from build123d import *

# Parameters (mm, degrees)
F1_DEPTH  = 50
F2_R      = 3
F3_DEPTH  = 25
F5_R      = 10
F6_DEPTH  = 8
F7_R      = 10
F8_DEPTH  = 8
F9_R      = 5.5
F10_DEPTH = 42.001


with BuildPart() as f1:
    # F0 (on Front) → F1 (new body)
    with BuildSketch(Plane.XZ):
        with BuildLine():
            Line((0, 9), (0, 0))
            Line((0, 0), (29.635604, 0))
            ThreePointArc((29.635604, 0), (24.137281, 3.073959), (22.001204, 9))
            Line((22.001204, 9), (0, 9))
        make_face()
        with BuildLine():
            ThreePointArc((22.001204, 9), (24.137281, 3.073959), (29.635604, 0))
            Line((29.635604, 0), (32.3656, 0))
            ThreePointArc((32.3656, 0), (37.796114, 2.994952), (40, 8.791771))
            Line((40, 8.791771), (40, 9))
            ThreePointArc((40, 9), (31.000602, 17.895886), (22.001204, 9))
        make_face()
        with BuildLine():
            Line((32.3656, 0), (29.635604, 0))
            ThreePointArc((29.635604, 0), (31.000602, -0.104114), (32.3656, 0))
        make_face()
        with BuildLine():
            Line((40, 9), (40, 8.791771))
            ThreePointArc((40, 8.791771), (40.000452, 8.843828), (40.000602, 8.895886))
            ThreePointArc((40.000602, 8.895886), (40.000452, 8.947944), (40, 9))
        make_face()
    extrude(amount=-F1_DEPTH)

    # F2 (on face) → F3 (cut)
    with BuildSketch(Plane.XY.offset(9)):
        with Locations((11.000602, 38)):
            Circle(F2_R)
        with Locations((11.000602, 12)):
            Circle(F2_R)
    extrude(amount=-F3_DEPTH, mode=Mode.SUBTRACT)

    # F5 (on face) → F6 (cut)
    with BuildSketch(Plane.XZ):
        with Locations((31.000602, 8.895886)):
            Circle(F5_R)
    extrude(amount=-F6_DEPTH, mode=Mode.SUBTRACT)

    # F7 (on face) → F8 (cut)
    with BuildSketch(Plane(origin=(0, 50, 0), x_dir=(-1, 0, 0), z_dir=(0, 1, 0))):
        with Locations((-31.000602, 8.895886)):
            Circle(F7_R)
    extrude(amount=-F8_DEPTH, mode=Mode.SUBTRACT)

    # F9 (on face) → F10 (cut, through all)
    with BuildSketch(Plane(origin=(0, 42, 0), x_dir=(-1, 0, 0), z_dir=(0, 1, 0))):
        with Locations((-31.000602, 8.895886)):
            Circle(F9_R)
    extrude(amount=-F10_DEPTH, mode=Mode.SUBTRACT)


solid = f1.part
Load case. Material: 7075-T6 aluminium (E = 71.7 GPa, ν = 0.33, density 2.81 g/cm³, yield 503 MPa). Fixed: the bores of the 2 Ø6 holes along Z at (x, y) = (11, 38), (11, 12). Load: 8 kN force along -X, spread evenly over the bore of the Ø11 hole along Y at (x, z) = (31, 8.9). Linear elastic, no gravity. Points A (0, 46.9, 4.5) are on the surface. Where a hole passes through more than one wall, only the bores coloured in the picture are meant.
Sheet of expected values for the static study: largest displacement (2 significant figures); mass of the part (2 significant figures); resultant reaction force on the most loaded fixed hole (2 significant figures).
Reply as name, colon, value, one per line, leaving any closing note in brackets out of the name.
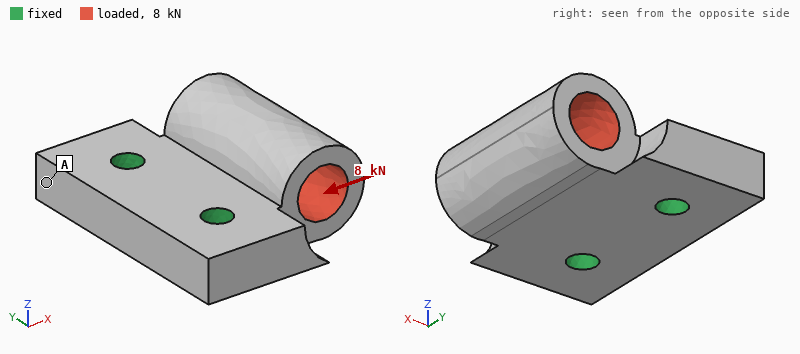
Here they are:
largest displacement: 0.11 mm
mass of the part: 43 g
resultant reaction force on the most loaded fixed hole: 4.1 kN
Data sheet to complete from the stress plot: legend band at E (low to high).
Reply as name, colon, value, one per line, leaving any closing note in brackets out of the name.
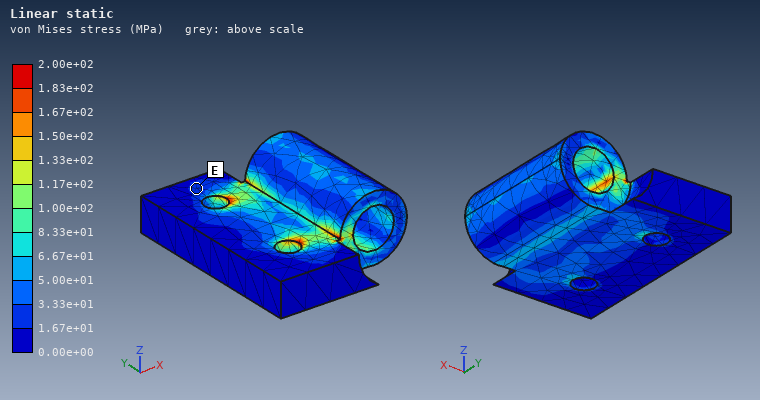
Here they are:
legend band at E: 1.67e+01 to 3.33e+01 MPa
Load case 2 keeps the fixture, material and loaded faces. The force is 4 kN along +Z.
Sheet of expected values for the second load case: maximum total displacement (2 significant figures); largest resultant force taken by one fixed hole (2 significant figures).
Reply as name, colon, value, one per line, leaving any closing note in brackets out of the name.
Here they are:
maximum total displacement: 0.14 mm
largest resultant force taken by one fixed hole: 2.0 kN
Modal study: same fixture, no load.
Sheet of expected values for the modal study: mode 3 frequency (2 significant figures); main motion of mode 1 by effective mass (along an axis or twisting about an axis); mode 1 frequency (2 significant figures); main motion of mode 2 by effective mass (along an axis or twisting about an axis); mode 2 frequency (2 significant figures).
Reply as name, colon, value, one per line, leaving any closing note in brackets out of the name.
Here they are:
mode 3 frequency: 21 kHz
main motion of mode 1 by effective mass: along Z
mode 1 frequency: 7400 Hz
main motion of mode 2 by effective mass: along Y
mode 2 frequency: 17 kHz
